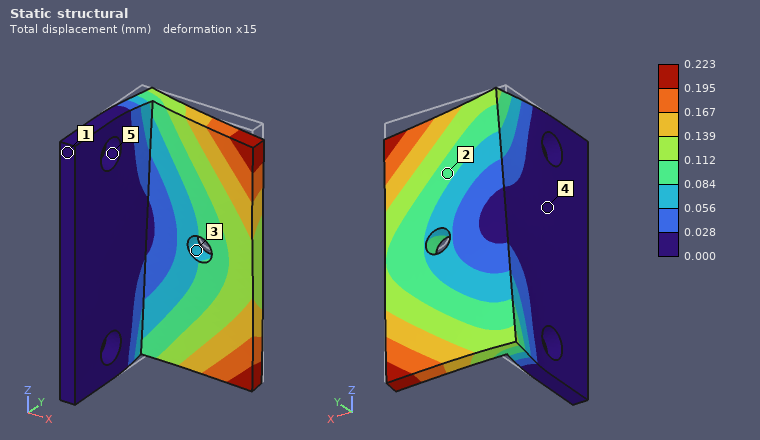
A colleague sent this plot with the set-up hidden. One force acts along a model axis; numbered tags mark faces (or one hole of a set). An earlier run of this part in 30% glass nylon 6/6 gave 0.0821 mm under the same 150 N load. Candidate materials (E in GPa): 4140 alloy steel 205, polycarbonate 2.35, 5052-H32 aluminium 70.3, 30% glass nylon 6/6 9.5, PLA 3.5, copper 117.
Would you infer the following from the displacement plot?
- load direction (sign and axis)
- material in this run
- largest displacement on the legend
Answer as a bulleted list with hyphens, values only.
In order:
- -Z
- PLA
- 0.223 mm
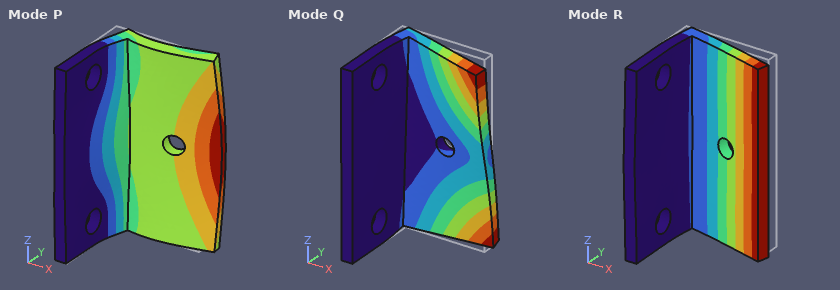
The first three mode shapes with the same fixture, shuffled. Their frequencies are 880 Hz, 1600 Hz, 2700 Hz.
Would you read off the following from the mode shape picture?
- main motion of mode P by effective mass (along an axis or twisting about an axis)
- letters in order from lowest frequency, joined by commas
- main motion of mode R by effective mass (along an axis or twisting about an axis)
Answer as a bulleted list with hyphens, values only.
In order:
- along X
- R, Q, P
- along Y
